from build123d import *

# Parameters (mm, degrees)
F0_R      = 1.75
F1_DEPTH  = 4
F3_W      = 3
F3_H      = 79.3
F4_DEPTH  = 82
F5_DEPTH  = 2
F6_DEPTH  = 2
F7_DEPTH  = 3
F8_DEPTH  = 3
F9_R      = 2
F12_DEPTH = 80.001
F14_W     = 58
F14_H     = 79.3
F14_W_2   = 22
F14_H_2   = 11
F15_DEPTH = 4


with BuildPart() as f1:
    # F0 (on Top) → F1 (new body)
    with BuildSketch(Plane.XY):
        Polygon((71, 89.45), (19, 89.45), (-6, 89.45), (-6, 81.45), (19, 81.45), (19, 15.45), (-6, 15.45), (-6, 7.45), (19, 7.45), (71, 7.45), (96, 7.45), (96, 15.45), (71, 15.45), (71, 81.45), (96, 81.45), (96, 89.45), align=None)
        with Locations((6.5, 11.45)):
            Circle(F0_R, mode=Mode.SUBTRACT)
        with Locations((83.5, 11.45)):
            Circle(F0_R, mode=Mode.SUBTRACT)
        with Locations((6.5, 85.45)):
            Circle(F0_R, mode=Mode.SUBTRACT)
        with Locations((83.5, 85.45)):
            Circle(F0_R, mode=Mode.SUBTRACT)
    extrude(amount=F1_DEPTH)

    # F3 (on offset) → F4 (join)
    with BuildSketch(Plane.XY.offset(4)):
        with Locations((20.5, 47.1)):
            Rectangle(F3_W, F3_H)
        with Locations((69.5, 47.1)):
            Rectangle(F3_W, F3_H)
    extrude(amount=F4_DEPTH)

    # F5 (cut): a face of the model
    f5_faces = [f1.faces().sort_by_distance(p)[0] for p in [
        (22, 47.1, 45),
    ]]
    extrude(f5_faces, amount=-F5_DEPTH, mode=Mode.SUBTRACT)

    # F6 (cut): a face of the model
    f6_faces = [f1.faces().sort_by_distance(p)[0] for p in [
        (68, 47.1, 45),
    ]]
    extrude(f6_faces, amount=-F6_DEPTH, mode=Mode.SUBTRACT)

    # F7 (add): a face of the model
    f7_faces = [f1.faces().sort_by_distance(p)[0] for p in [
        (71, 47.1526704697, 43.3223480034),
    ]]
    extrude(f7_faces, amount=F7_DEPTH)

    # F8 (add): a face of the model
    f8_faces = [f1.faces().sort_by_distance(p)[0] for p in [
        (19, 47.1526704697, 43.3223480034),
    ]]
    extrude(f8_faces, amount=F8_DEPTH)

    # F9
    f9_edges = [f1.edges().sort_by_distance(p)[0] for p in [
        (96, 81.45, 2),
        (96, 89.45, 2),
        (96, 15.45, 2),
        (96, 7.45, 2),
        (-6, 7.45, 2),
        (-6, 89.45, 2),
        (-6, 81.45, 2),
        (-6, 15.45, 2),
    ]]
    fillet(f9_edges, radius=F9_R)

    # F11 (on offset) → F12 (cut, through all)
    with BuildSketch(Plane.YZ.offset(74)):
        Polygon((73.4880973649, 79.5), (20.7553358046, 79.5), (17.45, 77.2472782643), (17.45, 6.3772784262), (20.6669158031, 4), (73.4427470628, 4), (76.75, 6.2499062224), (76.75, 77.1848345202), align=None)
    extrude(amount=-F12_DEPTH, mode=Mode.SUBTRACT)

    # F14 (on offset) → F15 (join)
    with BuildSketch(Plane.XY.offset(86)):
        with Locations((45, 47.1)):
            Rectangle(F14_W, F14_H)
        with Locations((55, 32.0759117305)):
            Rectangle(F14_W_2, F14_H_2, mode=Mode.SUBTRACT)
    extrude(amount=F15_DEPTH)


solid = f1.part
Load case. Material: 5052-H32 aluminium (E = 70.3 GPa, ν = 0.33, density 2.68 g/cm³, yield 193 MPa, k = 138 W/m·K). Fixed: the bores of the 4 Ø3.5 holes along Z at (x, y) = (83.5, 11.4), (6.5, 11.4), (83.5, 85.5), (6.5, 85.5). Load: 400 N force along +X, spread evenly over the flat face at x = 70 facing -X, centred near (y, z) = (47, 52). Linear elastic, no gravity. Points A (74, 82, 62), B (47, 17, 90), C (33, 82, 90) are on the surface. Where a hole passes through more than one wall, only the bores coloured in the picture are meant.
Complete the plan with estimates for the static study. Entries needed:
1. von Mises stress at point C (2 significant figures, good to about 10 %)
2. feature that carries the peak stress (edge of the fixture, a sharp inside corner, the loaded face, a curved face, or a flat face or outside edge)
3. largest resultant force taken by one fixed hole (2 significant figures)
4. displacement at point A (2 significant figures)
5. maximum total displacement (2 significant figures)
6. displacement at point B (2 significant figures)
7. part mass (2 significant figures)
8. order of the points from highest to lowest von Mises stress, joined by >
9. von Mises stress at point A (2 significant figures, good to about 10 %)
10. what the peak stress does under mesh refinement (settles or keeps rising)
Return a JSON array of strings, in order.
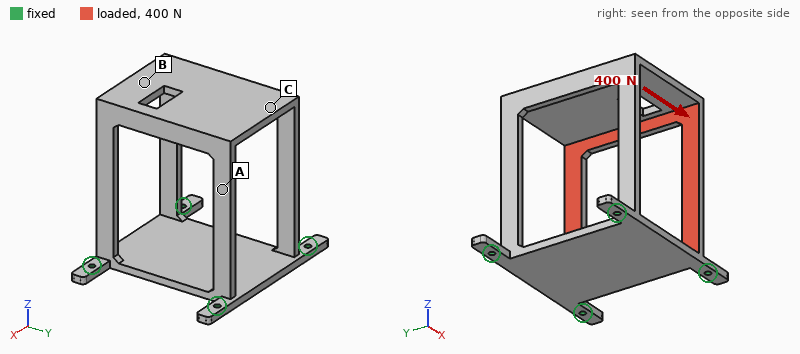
["17 MPa", "a sharp inside corner", "190 N", "0.74 mm", "0.86 mm", "0.85 mm", "150 g", "A > C > B", "53 MPa", "keeps rising"]
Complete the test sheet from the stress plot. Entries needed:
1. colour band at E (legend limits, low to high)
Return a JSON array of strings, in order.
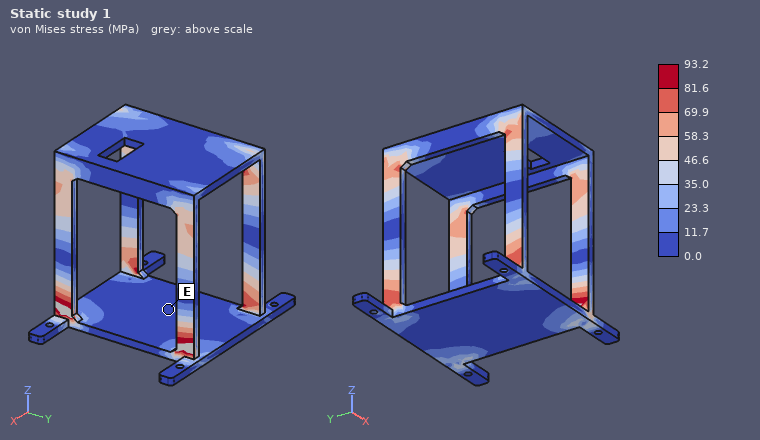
["0.0 to 11.7 MPa"]
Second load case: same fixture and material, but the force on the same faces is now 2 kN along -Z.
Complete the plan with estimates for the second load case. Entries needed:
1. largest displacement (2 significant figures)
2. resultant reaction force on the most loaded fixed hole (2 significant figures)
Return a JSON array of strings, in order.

["0.19 mm", "920 N"]
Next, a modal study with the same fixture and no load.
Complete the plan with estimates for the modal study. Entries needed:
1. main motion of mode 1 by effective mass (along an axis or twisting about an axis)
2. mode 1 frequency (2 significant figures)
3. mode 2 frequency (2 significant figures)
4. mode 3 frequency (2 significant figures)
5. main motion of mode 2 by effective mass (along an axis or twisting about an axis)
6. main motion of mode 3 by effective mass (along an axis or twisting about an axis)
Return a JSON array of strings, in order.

["along X", "320 Hz", "640 Hz", "680 Hz", "along Y", "twisting about Z"]
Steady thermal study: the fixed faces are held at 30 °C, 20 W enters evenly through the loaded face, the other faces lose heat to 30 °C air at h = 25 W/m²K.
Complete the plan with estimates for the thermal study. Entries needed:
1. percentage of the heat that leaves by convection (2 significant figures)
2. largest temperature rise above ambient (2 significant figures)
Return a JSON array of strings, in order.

["52 %", "32 K"]
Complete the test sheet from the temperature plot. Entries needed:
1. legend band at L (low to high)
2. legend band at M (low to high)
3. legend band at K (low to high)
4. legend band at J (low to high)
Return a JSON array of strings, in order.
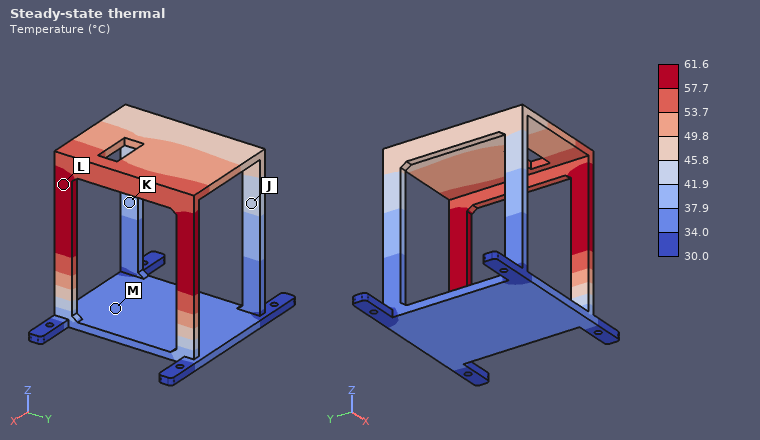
["57.7 to 61.6 °C", "34.0 to 37.9 °C", "37.9 to 41.9 °C", "41.9 to 45.8 °C"]
